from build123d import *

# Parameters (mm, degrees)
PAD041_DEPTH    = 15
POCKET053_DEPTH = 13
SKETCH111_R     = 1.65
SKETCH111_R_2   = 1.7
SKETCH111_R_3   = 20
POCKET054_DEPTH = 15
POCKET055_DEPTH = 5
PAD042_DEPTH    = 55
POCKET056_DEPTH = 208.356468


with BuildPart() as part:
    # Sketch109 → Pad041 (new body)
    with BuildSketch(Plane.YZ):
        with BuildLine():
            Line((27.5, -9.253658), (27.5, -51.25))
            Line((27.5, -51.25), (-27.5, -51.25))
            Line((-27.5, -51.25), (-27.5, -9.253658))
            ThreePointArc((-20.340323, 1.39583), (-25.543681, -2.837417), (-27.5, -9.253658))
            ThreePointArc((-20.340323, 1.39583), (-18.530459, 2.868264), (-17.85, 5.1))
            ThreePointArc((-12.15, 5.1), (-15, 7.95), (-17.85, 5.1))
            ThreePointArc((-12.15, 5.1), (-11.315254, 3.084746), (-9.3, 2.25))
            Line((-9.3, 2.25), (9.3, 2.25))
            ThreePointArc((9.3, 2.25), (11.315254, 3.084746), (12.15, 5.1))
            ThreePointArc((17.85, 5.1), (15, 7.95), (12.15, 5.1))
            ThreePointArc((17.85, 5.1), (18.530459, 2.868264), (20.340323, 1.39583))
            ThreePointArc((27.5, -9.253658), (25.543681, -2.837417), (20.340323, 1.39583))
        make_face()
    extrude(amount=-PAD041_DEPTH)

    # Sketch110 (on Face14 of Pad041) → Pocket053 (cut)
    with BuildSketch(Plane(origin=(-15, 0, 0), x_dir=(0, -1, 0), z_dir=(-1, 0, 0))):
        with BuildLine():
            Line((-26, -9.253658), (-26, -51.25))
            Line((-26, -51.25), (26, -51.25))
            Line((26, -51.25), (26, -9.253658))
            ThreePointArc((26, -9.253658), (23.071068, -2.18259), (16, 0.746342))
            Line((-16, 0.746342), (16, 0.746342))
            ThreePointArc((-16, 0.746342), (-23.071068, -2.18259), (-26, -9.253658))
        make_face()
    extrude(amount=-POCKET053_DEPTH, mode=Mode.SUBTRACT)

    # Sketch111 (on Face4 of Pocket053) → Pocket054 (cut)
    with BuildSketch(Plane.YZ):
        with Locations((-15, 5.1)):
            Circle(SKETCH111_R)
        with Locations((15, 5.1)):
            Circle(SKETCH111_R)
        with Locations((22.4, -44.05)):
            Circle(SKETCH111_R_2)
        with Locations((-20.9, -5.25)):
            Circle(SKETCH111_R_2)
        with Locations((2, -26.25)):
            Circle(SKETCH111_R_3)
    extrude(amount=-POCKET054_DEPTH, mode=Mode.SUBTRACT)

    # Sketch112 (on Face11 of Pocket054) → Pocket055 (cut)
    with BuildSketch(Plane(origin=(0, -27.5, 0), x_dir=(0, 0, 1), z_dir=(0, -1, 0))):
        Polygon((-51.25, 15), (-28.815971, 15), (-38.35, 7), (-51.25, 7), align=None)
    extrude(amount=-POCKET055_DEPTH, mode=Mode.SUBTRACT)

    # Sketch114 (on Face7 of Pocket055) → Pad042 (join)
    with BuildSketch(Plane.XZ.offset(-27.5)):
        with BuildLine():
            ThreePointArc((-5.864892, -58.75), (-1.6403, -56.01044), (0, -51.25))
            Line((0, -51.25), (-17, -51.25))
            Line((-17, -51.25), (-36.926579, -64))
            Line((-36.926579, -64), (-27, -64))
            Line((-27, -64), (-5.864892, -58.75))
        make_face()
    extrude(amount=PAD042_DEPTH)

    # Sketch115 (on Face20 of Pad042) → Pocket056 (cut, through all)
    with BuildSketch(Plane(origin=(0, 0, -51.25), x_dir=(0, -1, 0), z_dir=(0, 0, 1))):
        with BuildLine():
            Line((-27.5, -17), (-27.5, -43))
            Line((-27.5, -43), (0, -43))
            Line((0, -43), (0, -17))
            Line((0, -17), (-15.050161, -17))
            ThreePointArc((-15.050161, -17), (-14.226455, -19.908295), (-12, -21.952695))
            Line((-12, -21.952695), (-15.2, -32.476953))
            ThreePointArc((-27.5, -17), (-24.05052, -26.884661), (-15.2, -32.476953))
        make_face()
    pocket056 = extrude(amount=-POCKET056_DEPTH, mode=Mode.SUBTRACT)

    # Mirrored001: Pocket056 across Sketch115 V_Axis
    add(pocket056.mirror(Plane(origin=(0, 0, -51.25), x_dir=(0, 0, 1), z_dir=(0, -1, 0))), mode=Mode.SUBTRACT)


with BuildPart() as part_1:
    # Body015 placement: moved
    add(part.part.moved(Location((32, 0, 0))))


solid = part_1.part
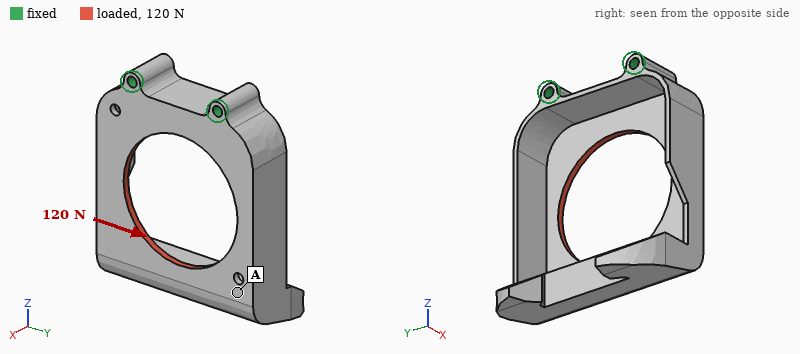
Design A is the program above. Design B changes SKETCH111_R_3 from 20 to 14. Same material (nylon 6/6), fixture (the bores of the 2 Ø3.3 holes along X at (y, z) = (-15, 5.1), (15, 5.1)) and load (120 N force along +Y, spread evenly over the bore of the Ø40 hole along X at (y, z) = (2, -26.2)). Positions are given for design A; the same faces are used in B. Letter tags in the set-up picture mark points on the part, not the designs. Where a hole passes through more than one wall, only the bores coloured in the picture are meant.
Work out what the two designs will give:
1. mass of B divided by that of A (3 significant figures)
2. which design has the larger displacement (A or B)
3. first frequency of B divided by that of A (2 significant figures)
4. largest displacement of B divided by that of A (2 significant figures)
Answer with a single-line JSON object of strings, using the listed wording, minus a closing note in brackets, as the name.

{"mass of B divided by that of A": "1.08", "which design has the larger displacement": "A", "first frequency of B divided by that of A": "1.0", "largest displacement of B divided by that of A": "0.43"}
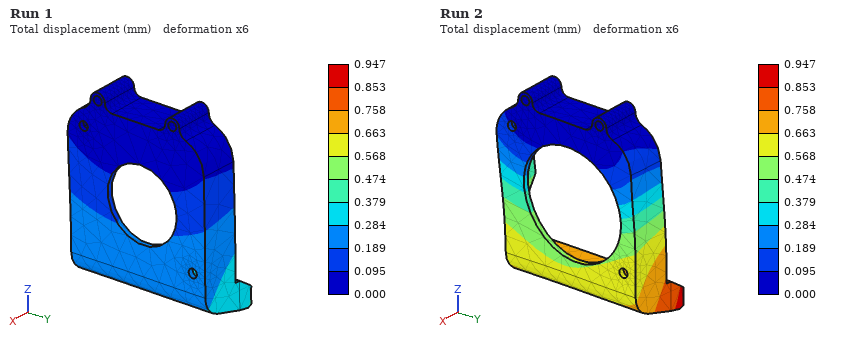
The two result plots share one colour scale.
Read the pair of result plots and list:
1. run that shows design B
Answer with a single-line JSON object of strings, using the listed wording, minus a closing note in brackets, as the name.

{"run that shows design B": "Run 1"}
